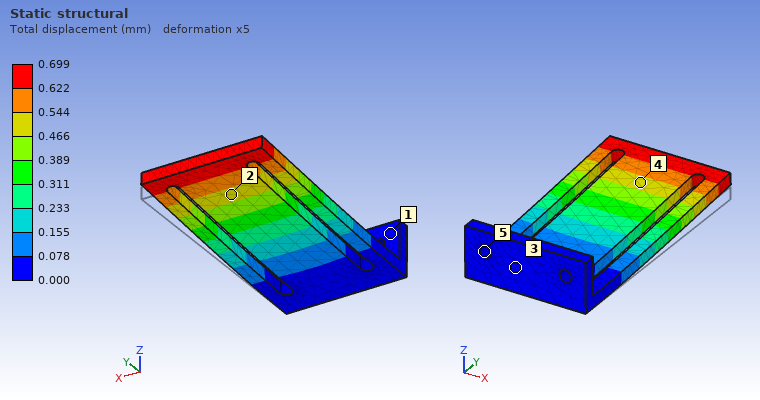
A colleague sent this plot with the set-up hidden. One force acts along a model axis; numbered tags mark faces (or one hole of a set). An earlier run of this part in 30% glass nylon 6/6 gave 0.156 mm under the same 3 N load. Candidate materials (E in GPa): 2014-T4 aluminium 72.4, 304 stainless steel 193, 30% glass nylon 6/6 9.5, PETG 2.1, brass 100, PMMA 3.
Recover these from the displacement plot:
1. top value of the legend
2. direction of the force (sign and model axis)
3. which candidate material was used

0.699 mm
+Z
PETG
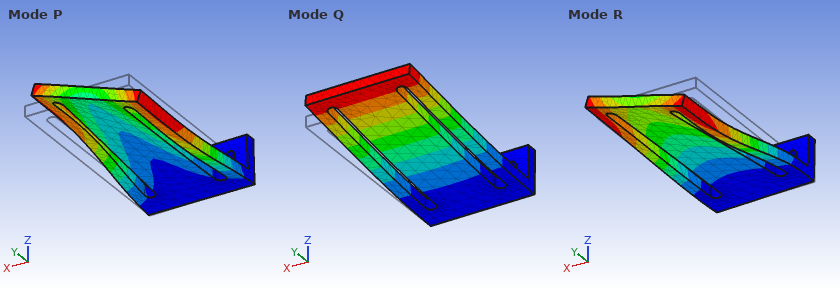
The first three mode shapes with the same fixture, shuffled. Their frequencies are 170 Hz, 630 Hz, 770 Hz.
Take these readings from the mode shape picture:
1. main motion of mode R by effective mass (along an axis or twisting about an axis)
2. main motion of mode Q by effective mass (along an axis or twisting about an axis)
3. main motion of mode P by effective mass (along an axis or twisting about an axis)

along X
along Z
along X
